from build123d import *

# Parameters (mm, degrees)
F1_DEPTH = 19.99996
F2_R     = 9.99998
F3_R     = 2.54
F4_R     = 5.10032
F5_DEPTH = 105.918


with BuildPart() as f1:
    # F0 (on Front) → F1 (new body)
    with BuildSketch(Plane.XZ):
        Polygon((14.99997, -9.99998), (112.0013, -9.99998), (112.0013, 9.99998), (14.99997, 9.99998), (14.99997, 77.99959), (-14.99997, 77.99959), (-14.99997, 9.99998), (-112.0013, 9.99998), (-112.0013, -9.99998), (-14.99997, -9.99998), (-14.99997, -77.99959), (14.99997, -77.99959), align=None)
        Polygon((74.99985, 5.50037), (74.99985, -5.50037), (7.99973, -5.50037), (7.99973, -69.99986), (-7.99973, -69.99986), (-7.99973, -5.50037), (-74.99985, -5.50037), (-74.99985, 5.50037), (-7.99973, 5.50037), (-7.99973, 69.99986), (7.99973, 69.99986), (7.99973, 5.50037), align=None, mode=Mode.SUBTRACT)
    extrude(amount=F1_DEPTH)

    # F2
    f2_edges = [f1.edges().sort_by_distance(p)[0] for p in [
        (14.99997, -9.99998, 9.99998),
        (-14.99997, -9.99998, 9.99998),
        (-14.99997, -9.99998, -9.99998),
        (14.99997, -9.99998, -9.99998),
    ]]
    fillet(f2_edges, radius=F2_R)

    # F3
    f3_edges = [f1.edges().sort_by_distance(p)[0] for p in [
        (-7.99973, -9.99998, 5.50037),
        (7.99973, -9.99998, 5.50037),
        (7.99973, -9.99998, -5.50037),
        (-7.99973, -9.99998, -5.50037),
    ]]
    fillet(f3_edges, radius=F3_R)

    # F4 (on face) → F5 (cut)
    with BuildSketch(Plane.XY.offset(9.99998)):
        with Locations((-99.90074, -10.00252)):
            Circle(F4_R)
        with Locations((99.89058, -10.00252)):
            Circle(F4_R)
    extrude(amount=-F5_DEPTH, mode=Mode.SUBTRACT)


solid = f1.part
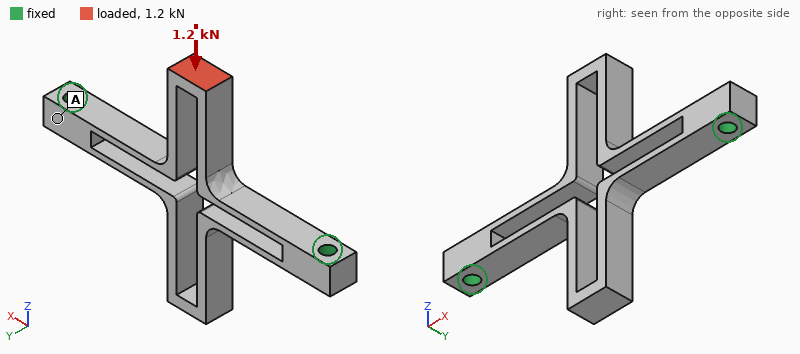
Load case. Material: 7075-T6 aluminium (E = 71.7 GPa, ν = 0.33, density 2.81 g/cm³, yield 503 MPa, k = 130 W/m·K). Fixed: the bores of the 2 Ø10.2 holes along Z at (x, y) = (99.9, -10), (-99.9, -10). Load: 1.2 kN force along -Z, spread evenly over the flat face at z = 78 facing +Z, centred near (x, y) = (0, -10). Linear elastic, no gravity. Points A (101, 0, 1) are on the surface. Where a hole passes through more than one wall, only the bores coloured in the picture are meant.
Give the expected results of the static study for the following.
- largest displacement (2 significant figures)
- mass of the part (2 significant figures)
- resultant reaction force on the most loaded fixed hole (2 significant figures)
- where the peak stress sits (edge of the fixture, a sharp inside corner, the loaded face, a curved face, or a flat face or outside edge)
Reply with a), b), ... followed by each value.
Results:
a) 1.2 mm
b) 270 g
c) 750 N
d) a flat face or outside edge
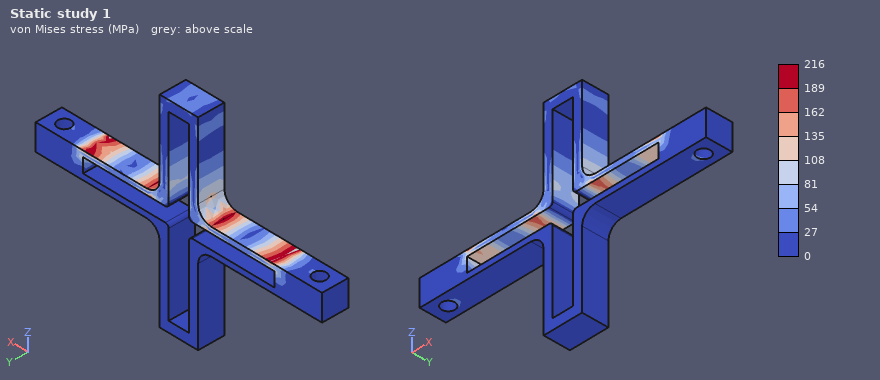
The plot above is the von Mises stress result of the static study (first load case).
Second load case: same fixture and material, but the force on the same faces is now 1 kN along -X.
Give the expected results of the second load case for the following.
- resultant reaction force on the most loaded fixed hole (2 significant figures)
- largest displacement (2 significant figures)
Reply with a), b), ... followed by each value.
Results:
a) 830 N
b) 2.0 mm
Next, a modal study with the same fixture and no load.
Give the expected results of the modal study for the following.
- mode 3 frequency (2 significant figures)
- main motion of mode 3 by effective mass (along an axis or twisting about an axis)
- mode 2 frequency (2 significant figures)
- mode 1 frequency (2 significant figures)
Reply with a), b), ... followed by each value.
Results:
a) 580 Hz
b) along Z
c) 330 Hz
d) 330 Hz
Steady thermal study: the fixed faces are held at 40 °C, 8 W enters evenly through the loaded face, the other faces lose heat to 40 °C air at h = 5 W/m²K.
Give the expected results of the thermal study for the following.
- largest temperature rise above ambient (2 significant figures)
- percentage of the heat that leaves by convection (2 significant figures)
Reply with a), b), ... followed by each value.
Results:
a) 32 K
b) 18 %
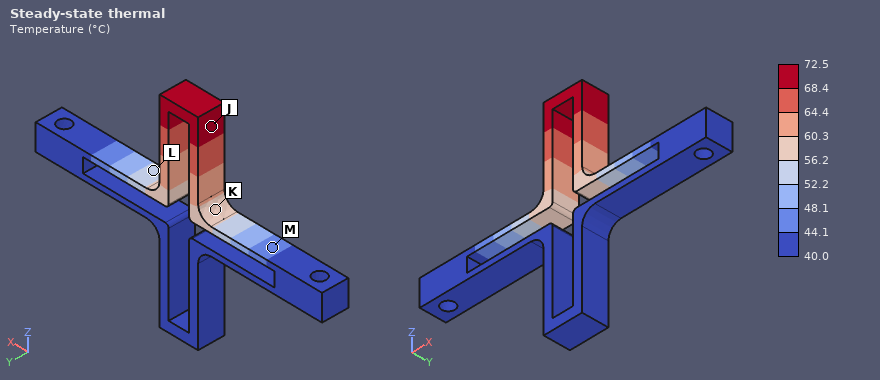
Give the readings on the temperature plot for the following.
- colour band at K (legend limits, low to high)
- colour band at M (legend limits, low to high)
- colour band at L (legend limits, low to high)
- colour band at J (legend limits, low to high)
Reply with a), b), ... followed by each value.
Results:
a) 56.2 to 60.3 °C
b) 44.1 to 48.1 °C
c) 52.2 to 56.2 °C
d) 68.4 to 72.5 °C
